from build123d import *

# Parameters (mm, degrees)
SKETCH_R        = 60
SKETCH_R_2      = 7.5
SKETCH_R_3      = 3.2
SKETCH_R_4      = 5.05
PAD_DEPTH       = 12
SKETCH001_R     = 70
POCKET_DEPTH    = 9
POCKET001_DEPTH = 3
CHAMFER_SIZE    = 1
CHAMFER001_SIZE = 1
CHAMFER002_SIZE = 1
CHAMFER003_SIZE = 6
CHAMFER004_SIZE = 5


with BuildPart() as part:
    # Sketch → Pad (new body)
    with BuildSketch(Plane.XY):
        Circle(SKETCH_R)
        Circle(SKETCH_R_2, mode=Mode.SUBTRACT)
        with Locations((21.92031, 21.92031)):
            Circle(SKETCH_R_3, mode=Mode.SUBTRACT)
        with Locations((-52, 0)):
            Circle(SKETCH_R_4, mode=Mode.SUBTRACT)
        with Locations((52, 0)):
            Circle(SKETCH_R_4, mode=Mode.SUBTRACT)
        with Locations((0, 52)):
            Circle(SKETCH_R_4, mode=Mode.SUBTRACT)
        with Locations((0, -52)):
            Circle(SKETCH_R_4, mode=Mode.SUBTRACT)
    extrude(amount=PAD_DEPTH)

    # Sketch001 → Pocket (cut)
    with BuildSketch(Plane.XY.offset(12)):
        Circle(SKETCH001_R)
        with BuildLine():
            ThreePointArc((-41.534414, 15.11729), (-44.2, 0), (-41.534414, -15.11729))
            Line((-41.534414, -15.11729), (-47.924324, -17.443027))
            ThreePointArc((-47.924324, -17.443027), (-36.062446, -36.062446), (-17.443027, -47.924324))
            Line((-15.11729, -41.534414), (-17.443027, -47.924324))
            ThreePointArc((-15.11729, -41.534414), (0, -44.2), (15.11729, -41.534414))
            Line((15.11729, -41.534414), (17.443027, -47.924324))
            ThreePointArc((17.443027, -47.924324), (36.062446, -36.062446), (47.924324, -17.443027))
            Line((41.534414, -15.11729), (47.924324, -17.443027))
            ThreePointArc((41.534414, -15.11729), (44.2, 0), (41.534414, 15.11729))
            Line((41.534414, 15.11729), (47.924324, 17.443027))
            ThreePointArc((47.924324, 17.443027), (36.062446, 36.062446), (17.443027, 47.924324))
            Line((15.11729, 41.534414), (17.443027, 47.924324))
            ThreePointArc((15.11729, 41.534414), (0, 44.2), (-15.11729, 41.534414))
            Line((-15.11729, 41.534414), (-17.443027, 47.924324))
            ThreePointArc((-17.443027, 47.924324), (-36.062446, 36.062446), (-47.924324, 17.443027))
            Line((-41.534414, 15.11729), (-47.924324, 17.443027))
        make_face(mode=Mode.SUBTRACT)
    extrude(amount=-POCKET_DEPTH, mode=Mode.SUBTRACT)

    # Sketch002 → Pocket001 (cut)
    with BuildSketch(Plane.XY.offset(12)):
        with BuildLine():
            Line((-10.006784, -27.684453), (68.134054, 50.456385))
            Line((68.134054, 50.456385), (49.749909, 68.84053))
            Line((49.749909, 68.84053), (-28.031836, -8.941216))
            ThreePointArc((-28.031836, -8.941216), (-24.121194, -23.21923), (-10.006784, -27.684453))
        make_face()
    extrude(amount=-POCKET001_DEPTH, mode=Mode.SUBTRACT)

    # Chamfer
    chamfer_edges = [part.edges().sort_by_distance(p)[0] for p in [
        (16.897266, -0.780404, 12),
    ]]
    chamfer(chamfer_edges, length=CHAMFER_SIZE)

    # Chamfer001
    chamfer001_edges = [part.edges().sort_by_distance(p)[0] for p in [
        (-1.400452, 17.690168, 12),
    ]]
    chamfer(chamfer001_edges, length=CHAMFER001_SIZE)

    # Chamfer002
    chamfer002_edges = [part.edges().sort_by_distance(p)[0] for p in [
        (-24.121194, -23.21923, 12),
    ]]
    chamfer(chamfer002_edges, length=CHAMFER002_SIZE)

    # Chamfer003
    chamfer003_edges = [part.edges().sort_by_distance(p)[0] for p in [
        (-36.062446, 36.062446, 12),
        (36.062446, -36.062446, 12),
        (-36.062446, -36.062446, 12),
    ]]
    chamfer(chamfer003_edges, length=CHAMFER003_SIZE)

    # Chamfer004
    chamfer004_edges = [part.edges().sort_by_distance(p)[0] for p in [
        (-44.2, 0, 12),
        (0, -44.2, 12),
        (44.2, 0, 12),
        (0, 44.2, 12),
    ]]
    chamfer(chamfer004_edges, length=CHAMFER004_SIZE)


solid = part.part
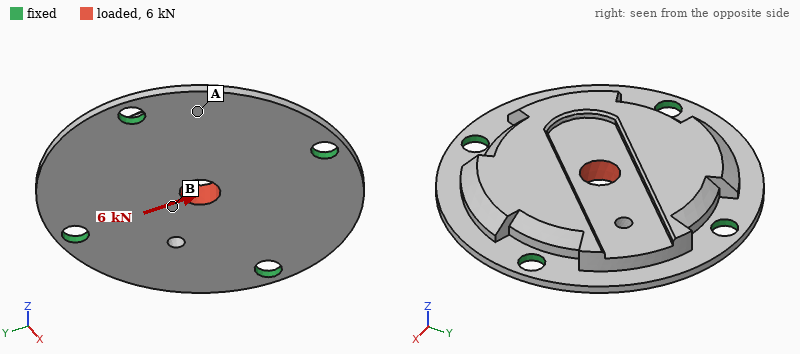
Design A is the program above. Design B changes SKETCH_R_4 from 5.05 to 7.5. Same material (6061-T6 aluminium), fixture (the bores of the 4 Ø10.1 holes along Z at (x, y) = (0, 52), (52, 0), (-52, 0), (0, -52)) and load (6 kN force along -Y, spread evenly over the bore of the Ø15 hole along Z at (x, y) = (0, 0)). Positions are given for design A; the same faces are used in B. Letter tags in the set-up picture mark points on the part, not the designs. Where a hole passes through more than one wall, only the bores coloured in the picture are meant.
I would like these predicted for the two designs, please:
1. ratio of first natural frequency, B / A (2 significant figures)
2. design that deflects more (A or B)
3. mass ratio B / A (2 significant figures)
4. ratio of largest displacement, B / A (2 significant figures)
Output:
1.2
A
0.99
0.86
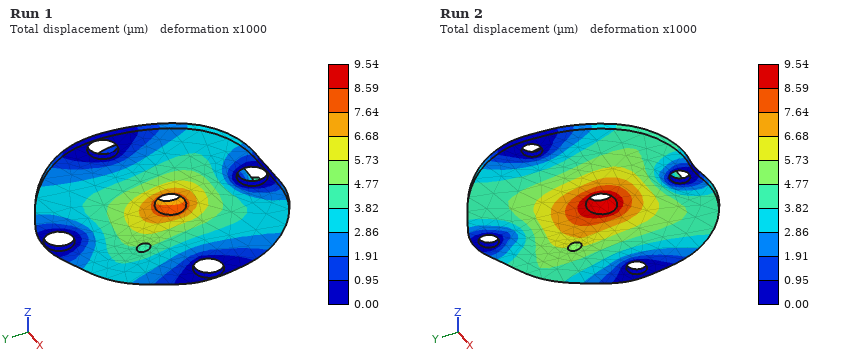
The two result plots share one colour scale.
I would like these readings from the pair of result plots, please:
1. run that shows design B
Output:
Run 1
